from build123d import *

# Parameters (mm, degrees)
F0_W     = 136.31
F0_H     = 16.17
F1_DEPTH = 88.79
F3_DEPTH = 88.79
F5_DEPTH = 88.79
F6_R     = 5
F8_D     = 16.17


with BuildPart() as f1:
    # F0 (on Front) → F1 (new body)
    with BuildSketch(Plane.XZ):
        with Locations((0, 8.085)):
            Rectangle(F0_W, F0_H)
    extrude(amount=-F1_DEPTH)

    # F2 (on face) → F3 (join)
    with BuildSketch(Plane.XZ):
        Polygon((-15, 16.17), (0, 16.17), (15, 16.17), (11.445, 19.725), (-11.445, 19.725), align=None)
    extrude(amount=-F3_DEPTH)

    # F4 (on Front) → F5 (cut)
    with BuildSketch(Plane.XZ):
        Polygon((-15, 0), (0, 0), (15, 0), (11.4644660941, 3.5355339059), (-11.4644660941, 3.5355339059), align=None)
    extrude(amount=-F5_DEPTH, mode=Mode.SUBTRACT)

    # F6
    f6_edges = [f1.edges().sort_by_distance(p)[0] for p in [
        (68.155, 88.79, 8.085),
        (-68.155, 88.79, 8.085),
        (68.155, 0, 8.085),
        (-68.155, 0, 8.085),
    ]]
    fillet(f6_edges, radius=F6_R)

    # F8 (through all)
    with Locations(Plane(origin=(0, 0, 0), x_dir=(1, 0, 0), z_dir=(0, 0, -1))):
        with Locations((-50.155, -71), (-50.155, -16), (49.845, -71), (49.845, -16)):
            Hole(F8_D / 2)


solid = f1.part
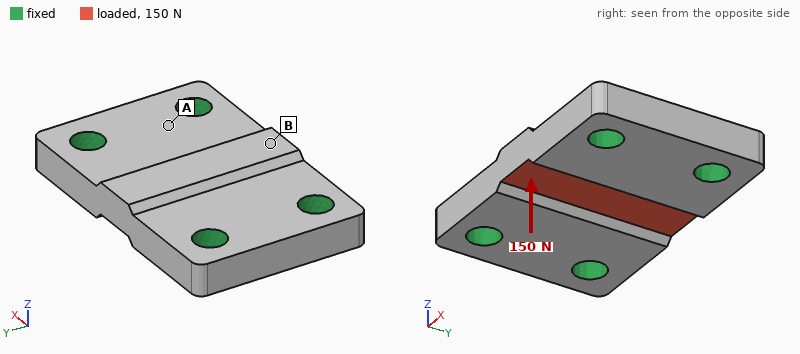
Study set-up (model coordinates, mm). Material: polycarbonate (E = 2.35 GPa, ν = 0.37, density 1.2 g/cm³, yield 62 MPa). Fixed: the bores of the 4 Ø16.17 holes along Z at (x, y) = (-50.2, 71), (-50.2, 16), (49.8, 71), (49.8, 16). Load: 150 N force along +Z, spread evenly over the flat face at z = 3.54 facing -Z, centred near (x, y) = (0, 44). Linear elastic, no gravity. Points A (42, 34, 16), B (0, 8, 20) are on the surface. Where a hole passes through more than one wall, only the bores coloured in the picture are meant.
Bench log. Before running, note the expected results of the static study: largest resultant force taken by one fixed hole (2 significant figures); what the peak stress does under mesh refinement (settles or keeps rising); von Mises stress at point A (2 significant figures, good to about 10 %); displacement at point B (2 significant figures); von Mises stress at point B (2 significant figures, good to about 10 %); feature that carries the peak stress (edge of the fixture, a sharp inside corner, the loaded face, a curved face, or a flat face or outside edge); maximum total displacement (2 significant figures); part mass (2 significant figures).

44 N
keeps rising
0.14 MPa
10 µm
0.32 MPa
edge of the fixture
11 µm
220 g
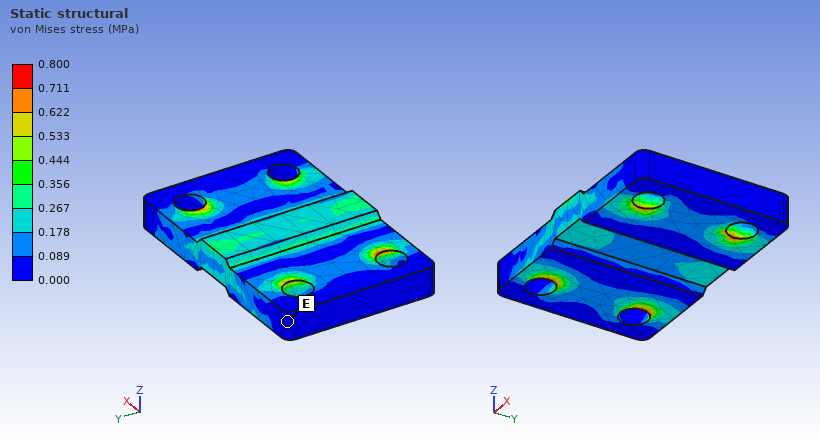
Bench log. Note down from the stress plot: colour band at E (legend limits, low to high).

0.000 to 0.089 MPa
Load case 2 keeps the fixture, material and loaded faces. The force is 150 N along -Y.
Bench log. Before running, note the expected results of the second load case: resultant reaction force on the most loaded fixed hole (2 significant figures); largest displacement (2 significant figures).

44 N
5.2 µm
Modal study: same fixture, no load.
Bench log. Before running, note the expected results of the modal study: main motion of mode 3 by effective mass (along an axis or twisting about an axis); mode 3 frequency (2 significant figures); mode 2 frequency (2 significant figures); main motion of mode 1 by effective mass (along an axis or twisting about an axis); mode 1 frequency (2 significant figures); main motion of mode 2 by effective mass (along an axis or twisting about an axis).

along Y
4100 Hz
2700 Hz
along Z
2300 Hz
twisting about X
